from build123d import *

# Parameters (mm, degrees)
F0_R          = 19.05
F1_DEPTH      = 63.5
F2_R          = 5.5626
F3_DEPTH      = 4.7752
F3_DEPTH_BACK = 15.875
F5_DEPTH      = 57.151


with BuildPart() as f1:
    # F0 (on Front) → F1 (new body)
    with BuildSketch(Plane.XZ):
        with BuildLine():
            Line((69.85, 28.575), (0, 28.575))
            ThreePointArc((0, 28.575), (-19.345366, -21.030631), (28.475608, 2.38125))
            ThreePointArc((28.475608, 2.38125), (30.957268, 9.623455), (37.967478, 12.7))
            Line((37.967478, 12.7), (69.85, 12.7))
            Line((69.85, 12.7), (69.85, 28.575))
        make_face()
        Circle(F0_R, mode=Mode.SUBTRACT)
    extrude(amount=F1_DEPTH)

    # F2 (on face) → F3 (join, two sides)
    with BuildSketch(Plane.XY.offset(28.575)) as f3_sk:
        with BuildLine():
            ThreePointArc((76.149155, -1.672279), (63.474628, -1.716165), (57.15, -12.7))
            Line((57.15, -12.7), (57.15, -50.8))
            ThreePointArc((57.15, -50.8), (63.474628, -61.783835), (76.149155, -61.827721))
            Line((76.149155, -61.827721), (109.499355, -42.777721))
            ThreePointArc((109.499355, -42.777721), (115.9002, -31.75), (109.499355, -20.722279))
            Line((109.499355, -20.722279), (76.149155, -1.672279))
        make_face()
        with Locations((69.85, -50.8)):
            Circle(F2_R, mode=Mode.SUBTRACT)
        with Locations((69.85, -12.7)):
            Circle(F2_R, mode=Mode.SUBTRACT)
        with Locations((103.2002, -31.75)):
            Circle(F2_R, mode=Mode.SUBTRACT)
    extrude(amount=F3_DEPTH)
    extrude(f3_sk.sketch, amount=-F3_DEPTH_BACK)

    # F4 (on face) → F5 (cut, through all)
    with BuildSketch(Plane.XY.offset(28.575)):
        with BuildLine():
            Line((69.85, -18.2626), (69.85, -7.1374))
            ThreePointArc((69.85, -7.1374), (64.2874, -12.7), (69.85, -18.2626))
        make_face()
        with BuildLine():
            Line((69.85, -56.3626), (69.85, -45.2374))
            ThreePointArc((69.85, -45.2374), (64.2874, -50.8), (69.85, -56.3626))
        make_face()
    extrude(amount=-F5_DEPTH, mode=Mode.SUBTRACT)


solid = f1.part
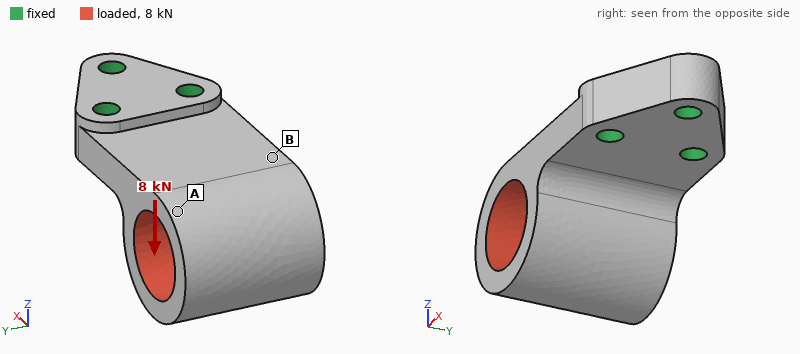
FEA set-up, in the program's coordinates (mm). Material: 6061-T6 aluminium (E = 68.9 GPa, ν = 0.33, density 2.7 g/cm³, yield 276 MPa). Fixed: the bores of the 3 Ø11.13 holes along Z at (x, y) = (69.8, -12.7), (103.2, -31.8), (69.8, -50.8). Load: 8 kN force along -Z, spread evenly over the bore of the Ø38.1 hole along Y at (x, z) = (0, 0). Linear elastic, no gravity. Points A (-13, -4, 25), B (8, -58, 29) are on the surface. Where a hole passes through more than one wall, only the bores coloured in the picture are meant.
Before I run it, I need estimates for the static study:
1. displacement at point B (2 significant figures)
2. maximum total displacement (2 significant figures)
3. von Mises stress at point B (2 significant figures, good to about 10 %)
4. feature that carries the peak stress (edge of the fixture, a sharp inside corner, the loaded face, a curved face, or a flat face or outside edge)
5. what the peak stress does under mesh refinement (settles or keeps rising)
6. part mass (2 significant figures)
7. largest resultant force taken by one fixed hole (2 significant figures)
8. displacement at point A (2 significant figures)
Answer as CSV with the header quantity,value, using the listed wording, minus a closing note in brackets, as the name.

quantity,value
displacement at point B,0.40 mm
maximum total displacement,0.84 mm
von Mises stress at point B,40 MPa
feature that carries the peak stress,edge of the fixture
what the peak stress does under mesh refinement,keeps rising
part mass,490 g
largest resultant force taken by one fixed hole,5.0 kN
displacement at point A,0.64 mm
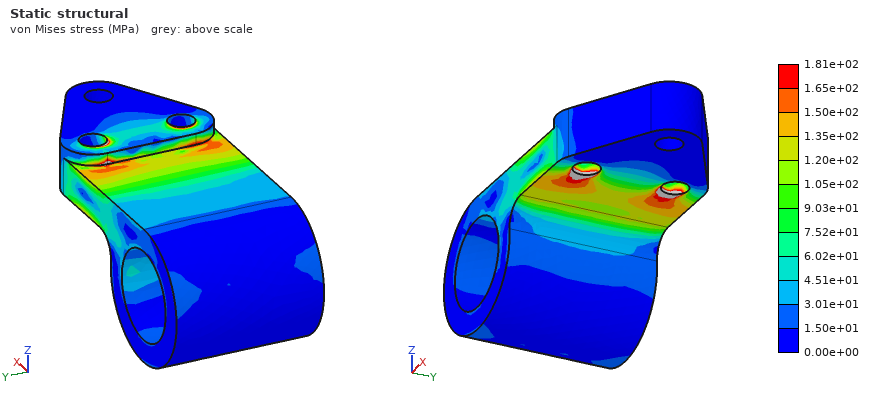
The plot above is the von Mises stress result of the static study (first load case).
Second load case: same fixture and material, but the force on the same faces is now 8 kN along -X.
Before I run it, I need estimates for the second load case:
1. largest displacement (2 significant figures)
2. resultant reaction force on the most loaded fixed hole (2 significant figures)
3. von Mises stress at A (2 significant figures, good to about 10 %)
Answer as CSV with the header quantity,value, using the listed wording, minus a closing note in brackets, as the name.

quantity,value
largest displacement,0.39 mm
resultant reaction force on the most loaded fixed hole,3.8 kN
von Mises stress at A,9.1 MPa
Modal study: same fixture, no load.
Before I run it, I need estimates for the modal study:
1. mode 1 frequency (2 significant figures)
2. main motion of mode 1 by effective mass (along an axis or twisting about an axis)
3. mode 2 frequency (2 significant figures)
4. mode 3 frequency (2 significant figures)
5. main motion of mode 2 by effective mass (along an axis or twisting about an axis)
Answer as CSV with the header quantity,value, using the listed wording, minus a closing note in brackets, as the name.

quantity,value
mode 1 frequency,1000 Hz
main motion of mode 1 by effective mass,along Z
mode 2 frequency,2500 Hz
mode 3 frequency,4300 Hz
main motion of mode 2 by effective mass,along Y
